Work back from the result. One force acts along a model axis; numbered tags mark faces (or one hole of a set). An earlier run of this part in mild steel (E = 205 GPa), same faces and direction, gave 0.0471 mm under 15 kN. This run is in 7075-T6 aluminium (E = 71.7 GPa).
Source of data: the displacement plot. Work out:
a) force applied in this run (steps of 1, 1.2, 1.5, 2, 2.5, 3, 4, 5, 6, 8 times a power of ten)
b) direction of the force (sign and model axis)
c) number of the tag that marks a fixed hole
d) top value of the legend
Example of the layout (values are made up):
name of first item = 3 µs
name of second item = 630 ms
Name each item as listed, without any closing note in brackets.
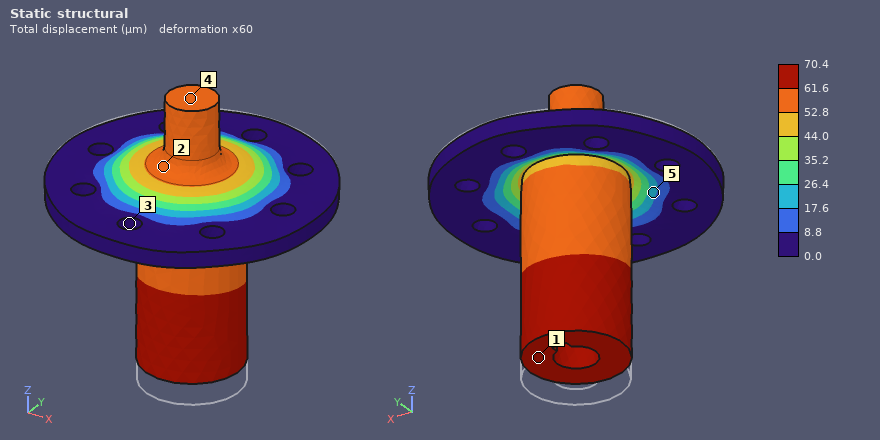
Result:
force applied in this run = 8 kN
direction of the force = +Z
number of the tag that marks a fixed hole = 3
top value of the legend = 70.4 µm
